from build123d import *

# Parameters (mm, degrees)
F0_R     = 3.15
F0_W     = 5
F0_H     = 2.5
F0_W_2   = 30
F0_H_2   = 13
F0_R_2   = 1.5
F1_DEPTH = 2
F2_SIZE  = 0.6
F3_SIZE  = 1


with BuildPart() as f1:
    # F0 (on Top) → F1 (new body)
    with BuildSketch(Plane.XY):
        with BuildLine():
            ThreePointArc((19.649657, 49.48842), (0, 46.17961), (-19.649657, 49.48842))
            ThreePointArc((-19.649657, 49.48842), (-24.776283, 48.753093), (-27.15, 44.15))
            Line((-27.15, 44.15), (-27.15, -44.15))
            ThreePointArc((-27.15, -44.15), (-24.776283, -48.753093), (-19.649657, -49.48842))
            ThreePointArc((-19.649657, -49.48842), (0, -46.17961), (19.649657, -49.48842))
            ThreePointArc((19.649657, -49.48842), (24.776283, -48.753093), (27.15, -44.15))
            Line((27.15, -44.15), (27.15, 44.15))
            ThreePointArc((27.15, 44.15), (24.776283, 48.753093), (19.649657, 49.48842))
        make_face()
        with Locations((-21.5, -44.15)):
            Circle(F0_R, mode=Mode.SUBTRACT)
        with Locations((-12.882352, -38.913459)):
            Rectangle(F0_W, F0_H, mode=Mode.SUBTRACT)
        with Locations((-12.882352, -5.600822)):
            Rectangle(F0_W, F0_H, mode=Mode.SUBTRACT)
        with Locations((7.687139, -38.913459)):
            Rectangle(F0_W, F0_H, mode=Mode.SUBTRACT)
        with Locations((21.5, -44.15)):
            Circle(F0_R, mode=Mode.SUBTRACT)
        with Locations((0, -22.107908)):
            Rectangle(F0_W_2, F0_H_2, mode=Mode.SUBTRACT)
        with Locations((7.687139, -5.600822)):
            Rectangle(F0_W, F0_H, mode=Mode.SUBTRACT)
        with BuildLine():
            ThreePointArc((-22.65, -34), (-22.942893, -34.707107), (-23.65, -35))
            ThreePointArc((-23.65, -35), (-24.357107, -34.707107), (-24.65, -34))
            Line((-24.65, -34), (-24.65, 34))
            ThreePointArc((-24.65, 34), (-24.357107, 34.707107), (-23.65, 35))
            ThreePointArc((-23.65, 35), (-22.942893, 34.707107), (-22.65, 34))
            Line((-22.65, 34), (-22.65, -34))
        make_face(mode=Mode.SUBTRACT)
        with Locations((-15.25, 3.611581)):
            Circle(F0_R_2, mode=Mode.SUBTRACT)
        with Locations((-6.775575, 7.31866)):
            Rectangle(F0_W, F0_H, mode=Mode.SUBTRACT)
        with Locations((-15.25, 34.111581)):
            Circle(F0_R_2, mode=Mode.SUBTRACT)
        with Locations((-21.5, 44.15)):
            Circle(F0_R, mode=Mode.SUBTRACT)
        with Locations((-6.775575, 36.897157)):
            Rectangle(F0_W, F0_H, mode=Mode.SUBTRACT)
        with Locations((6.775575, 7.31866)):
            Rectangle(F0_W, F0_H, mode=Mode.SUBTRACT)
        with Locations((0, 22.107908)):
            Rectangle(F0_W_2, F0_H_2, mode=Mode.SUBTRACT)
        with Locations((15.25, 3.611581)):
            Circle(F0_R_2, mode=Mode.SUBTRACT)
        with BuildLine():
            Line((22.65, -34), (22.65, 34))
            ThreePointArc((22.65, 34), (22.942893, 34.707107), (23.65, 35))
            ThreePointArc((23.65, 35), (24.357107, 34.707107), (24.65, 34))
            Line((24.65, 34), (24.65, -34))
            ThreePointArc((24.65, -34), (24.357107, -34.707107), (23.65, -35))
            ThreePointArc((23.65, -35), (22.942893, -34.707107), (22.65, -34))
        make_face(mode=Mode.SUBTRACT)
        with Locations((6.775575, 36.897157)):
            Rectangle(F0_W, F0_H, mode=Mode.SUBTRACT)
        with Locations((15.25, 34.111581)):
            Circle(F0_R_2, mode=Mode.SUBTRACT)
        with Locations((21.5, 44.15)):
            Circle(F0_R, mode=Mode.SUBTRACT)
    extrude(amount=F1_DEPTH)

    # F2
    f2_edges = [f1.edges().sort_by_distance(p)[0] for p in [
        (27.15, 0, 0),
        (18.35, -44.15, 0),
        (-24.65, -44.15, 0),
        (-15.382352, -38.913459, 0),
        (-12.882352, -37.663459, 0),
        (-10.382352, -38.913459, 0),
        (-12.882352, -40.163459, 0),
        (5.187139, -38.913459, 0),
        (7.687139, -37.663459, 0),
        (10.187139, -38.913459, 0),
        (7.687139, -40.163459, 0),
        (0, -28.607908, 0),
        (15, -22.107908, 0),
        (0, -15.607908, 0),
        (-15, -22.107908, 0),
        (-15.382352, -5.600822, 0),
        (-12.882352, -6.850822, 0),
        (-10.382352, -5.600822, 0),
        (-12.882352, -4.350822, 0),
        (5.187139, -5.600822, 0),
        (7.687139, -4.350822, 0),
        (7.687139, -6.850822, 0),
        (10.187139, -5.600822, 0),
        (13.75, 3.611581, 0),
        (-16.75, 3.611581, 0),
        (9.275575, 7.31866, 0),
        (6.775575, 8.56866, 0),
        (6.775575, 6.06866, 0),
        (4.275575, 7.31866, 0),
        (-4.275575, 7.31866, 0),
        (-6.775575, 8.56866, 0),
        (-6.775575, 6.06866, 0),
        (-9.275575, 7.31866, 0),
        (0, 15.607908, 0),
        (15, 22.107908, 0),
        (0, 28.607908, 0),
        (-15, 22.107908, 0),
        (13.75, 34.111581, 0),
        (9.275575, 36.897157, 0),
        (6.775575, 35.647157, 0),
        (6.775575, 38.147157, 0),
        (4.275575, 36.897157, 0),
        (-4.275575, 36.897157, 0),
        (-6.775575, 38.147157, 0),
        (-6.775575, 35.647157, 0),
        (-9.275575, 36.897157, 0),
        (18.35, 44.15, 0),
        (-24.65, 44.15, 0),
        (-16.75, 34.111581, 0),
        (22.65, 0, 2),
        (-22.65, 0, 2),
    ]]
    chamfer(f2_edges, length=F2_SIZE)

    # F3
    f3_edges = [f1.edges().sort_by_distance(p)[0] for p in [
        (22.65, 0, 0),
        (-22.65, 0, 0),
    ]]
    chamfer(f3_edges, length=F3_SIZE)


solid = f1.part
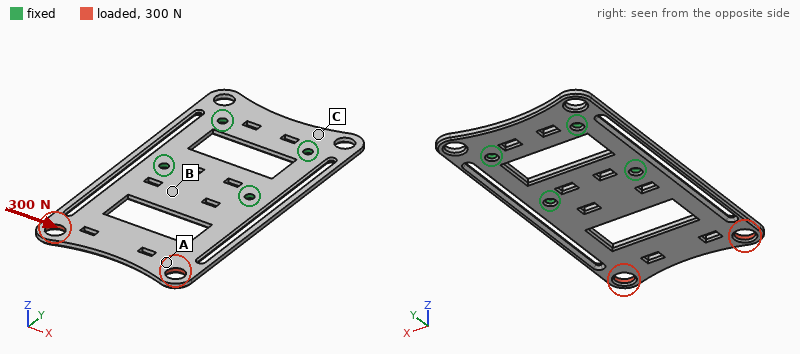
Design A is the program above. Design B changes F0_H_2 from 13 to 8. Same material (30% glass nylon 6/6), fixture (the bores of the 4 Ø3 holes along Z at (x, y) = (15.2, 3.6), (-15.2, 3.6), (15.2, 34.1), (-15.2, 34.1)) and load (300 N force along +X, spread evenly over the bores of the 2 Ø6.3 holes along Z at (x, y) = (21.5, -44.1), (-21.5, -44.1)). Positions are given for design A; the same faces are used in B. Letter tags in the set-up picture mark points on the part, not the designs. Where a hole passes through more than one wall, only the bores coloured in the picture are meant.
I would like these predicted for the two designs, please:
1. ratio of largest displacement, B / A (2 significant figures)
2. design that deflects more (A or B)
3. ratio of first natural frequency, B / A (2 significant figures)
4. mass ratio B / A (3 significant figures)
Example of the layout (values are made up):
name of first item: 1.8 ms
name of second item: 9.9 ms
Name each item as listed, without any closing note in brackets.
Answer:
ratio of largest displacement, B / A: 0.79
design that deflects more: A
ratio of first natural frequency, B / A: 1.0
mass ratio B / A: 1.08
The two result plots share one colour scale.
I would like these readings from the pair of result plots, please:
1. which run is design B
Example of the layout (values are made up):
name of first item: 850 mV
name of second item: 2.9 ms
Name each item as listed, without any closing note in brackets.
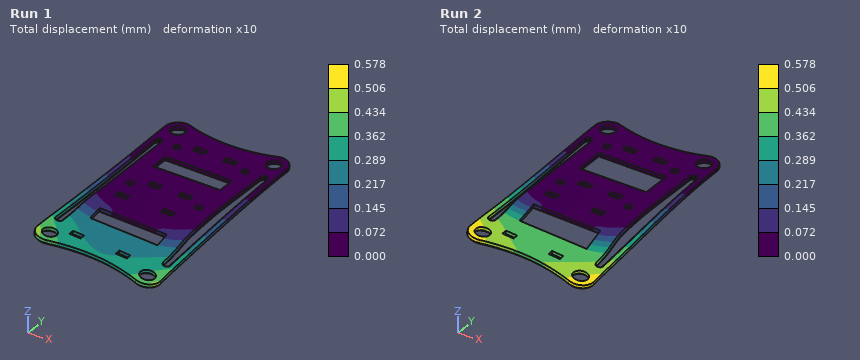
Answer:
which run is design B: Run 1
